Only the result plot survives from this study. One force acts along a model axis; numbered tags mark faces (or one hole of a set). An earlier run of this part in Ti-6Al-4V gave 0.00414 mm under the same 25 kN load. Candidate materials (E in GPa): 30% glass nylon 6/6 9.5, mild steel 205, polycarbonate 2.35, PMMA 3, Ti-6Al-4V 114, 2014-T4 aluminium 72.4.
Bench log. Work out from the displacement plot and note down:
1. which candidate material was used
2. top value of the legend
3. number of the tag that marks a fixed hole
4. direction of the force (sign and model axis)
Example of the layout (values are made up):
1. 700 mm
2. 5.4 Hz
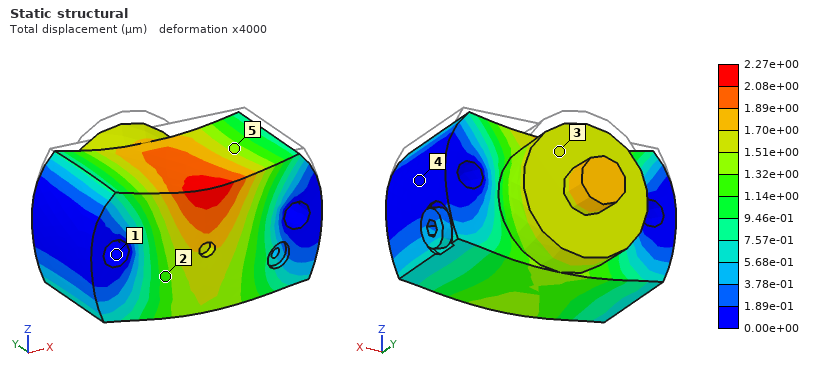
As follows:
1. mild steel
2. 2.27e+00 µm
3. 1
4. -Z
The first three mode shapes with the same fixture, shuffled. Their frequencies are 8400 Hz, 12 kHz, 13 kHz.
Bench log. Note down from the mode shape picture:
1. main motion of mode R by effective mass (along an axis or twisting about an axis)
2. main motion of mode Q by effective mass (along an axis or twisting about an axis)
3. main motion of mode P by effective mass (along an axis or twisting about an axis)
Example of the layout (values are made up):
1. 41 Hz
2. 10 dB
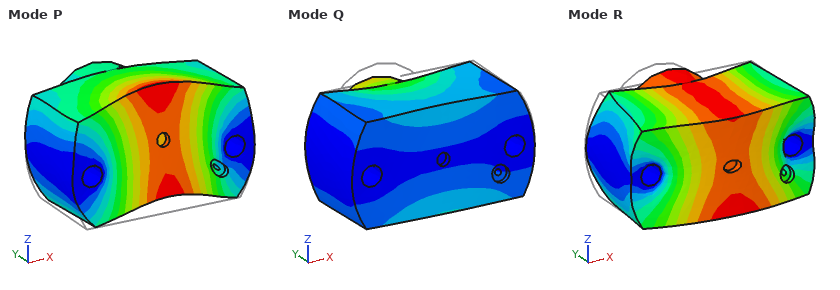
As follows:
1. along Y
2. along Z
3. along Z
